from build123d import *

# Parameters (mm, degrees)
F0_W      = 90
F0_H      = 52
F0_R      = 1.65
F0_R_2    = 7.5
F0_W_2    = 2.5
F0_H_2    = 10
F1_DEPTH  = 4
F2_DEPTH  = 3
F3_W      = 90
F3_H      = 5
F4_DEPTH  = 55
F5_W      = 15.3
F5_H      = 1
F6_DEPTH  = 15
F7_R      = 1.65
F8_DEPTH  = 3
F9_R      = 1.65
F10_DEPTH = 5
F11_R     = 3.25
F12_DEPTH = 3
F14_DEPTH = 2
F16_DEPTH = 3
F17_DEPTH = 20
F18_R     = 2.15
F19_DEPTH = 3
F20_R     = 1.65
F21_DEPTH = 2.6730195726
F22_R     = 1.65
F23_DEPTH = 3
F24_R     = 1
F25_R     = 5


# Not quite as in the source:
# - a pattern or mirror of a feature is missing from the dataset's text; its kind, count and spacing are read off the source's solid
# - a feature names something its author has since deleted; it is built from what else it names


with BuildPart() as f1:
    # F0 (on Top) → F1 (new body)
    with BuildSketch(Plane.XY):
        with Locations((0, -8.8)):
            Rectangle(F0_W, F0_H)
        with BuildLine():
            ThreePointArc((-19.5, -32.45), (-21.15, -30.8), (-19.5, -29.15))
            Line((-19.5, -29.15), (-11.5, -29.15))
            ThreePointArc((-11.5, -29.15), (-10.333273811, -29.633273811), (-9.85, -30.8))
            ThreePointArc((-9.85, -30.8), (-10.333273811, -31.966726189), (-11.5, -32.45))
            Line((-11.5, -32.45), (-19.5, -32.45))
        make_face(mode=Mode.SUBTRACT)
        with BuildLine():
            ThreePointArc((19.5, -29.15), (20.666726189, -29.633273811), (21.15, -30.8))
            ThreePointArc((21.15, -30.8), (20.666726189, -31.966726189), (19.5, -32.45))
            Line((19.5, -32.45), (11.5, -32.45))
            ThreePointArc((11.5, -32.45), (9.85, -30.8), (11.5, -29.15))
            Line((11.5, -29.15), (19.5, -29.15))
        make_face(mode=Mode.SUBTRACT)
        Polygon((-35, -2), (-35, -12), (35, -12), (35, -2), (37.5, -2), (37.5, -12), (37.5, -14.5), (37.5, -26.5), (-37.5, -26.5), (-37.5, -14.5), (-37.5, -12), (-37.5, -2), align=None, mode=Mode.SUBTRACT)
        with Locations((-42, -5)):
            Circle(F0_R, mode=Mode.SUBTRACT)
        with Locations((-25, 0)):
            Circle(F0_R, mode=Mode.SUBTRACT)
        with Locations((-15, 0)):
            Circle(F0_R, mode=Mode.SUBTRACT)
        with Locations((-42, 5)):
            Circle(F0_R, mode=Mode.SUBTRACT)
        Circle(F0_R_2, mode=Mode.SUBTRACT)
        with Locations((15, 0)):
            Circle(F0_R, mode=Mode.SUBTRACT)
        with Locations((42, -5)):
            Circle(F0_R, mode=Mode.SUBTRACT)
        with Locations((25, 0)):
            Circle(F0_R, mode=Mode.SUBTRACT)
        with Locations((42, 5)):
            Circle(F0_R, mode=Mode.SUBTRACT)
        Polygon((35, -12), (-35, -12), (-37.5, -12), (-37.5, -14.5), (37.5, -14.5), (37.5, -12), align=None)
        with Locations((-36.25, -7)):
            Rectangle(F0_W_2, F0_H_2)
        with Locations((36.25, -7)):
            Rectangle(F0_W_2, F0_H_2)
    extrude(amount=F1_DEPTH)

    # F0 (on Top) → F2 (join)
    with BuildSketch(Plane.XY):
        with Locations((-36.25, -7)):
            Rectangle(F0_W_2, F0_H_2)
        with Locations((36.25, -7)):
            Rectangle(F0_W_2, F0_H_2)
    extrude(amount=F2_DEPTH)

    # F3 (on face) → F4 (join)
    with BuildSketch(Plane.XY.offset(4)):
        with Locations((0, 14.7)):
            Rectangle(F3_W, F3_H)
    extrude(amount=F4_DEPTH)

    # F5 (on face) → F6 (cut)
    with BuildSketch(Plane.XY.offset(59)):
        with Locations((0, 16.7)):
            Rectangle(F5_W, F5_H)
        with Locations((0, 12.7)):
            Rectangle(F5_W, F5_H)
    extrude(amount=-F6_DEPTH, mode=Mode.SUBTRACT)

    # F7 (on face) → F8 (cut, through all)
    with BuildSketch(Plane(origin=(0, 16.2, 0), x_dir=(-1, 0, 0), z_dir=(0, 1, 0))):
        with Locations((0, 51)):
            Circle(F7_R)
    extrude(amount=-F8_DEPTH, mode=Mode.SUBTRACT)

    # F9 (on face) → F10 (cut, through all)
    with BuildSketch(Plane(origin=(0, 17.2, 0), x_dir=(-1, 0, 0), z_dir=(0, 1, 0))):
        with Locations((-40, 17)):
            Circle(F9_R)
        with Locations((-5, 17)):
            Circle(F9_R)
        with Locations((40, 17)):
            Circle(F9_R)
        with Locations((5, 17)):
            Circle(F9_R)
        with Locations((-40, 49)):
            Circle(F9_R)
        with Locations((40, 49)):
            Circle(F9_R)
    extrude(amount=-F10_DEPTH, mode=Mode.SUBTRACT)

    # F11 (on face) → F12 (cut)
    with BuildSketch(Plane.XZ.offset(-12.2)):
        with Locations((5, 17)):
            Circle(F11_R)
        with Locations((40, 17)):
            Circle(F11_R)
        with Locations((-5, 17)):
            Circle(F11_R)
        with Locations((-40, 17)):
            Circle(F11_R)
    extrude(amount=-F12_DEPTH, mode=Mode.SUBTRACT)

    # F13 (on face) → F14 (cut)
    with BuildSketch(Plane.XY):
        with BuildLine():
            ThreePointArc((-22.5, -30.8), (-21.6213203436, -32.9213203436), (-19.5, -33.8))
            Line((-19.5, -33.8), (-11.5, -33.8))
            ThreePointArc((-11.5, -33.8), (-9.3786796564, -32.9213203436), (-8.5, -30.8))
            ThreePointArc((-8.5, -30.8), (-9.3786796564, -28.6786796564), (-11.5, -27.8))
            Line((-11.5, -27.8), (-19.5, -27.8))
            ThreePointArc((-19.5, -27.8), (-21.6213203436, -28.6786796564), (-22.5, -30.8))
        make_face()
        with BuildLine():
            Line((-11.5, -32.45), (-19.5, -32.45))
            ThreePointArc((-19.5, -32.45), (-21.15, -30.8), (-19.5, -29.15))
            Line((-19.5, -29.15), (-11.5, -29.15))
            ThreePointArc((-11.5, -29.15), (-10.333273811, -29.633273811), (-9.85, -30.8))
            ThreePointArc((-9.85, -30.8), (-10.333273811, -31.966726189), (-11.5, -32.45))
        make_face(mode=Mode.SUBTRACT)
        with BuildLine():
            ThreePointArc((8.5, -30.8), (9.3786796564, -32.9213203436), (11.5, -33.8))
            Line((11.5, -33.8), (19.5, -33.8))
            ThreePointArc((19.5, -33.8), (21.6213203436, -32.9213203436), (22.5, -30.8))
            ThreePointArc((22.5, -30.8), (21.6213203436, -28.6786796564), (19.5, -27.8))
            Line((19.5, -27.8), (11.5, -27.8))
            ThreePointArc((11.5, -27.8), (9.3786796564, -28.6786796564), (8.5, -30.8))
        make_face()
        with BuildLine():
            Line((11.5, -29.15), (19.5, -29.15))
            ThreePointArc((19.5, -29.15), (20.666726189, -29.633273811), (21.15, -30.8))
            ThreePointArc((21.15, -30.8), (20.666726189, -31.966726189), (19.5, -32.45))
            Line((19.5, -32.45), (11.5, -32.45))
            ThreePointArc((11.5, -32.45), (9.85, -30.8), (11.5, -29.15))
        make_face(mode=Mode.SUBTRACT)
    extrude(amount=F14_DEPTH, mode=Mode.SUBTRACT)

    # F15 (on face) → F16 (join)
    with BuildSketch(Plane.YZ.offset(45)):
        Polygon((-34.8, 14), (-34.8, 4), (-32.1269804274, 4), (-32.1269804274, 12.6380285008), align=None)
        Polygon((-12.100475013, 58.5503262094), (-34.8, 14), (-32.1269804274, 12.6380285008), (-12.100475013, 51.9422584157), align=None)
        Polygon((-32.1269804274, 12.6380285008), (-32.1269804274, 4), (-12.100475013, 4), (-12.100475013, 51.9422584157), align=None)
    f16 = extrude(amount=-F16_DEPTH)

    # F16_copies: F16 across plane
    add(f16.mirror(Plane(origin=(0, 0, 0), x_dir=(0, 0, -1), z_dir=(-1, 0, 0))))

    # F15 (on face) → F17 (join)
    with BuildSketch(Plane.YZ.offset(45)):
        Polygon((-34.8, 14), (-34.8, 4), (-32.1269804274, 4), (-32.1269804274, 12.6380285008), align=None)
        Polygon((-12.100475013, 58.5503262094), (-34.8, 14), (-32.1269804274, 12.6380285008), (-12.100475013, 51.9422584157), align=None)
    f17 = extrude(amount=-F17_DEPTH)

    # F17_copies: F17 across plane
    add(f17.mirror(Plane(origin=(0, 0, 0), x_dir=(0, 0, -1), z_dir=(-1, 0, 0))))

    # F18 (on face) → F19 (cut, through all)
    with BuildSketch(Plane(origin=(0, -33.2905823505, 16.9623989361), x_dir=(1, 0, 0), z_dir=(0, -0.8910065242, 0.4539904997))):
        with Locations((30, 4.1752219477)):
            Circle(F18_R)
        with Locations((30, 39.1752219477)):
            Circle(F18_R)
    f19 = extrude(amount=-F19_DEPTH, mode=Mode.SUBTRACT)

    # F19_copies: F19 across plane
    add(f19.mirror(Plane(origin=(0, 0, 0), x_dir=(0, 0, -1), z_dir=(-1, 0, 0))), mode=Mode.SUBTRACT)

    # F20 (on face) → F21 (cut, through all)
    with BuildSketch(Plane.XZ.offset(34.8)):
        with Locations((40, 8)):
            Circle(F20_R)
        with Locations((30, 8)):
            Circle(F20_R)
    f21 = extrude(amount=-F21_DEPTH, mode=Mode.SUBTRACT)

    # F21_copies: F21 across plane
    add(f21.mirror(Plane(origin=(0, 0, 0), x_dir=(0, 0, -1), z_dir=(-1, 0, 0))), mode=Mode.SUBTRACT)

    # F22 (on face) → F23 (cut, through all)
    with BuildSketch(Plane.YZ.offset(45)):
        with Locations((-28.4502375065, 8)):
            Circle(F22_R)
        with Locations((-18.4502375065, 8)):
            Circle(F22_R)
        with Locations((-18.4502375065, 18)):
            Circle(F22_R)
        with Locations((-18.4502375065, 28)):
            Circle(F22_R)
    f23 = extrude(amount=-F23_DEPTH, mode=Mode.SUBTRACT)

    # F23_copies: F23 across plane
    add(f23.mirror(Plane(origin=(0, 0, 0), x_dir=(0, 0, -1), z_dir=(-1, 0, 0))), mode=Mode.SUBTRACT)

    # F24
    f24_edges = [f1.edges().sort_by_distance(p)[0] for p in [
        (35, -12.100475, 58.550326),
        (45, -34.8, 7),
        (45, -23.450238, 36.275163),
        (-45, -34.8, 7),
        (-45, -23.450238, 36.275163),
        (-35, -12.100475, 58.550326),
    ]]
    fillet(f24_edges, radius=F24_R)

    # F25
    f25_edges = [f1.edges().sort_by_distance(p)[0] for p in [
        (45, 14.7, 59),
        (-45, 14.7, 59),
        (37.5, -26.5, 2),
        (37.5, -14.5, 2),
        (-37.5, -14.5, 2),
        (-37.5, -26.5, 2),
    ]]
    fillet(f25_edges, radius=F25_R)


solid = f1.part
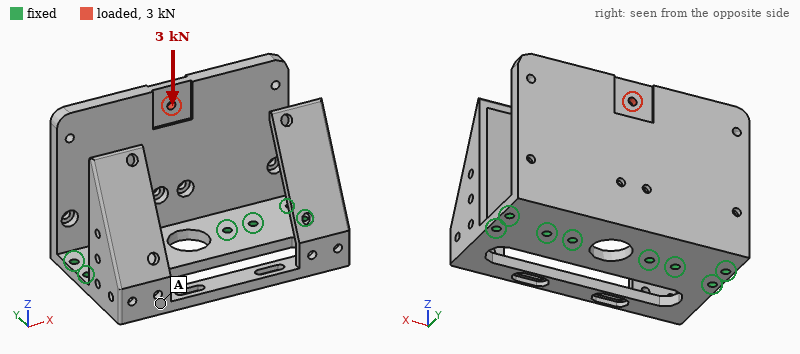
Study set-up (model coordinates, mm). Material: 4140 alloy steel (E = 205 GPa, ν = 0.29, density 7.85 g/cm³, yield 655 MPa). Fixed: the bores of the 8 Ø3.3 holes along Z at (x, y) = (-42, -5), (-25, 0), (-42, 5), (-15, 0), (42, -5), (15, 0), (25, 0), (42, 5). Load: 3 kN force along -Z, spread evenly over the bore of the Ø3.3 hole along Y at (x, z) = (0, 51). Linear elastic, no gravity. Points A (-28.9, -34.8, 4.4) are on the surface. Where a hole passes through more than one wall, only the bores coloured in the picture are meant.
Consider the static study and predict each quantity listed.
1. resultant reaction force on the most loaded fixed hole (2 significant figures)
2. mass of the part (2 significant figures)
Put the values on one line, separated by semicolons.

1.3 kN; 370 g
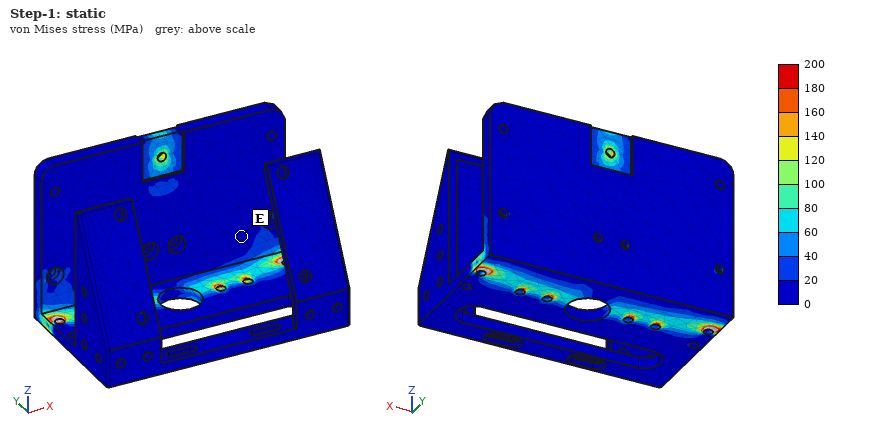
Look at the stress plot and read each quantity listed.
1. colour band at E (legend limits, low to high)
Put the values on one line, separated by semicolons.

0 to 20 MPa
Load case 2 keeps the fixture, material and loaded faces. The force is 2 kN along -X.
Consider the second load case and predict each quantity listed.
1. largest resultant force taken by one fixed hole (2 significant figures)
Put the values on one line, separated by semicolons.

1.3 kN
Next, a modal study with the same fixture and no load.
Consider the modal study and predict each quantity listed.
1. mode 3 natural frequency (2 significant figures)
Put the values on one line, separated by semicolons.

840 Hz
